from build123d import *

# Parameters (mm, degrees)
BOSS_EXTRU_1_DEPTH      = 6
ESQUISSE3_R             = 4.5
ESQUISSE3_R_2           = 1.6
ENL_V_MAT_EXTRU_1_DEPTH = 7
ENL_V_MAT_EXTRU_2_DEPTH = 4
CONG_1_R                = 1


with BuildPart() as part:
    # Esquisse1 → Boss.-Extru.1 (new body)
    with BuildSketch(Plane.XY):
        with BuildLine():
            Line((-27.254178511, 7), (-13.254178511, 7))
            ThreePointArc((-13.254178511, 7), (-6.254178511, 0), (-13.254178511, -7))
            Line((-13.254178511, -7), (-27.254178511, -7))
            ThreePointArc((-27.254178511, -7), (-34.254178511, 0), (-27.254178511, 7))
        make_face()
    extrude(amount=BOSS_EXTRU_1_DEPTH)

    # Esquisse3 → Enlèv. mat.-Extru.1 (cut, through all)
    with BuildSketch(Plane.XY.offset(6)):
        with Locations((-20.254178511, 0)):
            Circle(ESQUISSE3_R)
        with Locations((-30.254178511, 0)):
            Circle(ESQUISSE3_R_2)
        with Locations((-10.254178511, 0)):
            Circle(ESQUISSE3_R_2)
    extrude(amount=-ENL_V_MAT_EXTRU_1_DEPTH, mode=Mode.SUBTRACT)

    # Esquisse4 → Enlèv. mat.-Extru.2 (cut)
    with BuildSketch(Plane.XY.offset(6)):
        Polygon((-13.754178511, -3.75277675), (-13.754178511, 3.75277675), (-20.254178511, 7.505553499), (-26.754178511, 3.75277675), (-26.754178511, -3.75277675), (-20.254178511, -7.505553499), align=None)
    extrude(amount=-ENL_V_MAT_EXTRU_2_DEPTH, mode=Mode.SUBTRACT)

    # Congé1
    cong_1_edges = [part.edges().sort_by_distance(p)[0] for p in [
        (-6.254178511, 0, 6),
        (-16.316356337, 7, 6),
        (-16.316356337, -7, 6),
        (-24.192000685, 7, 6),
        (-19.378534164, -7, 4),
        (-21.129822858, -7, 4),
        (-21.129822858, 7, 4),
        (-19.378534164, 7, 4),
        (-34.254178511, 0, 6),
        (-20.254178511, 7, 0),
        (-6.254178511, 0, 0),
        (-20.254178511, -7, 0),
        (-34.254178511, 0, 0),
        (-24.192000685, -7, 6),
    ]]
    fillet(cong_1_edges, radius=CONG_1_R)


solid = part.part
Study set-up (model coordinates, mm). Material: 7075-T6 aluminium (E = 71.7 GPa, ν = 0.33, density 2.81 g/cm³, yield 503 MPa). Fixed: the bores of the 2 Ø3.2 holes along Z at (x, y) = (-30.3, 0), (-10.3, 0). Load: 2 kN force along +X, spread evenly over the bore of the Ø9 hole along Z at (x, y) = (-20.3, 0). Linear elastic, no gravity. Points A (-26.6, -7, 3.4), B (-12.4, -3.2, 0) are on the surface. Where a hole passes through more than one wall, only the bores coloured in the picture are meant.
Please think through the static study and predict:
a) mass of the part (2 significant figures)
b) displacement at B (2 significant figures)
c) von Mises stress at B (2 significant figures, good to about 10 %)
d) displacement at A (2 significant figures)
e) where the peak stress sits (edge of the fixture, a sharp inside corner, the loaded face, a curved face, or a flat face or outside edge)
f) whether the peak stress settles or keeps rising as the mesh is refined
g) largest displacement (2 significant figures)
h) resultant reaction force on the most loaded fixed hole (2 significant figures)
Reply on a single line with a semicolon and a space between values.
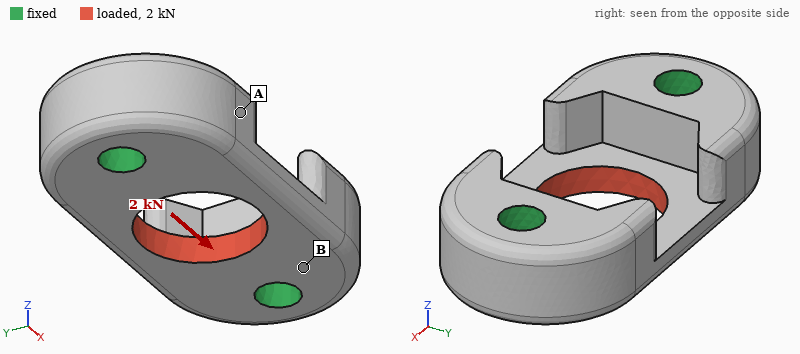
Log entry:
3.5 g; 2.4 µm; 35 MPa; 2.8 µm; edge of the fixture; keeps rising; 7.1 µm; 1.0 kN
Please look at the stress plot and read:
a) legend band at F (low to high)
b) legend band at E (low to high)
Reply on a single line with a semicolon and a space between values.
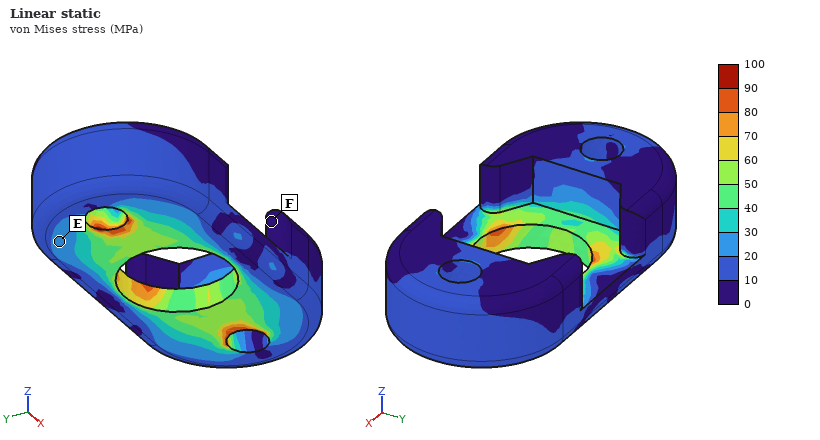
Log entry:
0 to 10 MPa; 20 to 30 MPa
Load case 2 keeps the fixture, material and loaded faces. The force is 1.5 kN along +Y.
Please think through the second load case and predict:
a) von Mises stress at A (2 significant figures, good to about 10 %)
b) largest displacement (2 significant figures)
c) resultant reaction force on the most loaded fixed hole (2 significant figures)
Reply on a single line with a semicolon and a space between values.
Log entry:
18 MPa; 14 µm; 750 N
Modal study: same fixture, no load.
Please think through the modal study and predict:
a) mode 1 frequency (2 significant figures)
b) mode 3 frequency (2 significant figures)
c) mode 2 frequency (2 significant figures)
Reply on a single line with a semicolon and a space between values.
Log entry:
53 kHz; 63 kHz; 55 kHz
